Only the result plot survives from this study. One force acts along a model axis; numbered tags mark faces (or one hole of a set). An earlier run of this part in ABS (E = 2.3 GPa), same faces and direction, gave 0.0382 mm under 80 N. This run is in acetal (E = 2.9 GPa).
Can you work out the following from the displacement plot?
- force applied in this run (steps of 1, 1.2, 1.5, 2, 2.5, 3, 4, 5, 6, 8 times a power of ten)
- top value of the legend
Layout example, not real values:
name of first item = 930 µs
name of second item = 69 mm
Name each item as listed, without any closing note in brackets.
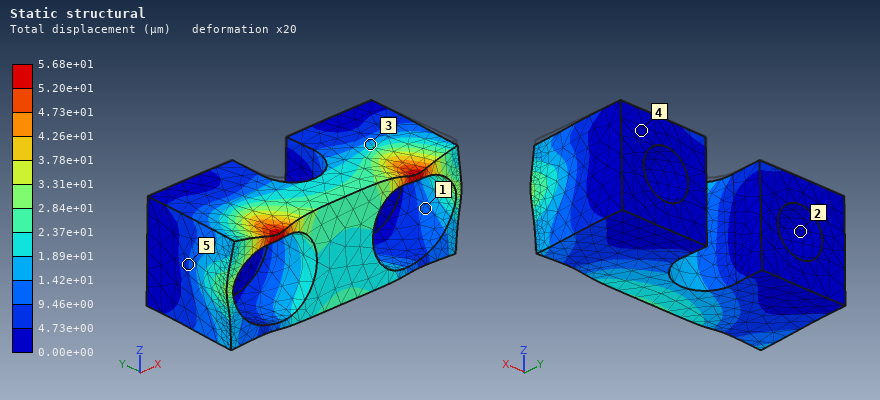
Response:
force applied in this run = 150 N
top value of the legend = 5.68e+01 µm
